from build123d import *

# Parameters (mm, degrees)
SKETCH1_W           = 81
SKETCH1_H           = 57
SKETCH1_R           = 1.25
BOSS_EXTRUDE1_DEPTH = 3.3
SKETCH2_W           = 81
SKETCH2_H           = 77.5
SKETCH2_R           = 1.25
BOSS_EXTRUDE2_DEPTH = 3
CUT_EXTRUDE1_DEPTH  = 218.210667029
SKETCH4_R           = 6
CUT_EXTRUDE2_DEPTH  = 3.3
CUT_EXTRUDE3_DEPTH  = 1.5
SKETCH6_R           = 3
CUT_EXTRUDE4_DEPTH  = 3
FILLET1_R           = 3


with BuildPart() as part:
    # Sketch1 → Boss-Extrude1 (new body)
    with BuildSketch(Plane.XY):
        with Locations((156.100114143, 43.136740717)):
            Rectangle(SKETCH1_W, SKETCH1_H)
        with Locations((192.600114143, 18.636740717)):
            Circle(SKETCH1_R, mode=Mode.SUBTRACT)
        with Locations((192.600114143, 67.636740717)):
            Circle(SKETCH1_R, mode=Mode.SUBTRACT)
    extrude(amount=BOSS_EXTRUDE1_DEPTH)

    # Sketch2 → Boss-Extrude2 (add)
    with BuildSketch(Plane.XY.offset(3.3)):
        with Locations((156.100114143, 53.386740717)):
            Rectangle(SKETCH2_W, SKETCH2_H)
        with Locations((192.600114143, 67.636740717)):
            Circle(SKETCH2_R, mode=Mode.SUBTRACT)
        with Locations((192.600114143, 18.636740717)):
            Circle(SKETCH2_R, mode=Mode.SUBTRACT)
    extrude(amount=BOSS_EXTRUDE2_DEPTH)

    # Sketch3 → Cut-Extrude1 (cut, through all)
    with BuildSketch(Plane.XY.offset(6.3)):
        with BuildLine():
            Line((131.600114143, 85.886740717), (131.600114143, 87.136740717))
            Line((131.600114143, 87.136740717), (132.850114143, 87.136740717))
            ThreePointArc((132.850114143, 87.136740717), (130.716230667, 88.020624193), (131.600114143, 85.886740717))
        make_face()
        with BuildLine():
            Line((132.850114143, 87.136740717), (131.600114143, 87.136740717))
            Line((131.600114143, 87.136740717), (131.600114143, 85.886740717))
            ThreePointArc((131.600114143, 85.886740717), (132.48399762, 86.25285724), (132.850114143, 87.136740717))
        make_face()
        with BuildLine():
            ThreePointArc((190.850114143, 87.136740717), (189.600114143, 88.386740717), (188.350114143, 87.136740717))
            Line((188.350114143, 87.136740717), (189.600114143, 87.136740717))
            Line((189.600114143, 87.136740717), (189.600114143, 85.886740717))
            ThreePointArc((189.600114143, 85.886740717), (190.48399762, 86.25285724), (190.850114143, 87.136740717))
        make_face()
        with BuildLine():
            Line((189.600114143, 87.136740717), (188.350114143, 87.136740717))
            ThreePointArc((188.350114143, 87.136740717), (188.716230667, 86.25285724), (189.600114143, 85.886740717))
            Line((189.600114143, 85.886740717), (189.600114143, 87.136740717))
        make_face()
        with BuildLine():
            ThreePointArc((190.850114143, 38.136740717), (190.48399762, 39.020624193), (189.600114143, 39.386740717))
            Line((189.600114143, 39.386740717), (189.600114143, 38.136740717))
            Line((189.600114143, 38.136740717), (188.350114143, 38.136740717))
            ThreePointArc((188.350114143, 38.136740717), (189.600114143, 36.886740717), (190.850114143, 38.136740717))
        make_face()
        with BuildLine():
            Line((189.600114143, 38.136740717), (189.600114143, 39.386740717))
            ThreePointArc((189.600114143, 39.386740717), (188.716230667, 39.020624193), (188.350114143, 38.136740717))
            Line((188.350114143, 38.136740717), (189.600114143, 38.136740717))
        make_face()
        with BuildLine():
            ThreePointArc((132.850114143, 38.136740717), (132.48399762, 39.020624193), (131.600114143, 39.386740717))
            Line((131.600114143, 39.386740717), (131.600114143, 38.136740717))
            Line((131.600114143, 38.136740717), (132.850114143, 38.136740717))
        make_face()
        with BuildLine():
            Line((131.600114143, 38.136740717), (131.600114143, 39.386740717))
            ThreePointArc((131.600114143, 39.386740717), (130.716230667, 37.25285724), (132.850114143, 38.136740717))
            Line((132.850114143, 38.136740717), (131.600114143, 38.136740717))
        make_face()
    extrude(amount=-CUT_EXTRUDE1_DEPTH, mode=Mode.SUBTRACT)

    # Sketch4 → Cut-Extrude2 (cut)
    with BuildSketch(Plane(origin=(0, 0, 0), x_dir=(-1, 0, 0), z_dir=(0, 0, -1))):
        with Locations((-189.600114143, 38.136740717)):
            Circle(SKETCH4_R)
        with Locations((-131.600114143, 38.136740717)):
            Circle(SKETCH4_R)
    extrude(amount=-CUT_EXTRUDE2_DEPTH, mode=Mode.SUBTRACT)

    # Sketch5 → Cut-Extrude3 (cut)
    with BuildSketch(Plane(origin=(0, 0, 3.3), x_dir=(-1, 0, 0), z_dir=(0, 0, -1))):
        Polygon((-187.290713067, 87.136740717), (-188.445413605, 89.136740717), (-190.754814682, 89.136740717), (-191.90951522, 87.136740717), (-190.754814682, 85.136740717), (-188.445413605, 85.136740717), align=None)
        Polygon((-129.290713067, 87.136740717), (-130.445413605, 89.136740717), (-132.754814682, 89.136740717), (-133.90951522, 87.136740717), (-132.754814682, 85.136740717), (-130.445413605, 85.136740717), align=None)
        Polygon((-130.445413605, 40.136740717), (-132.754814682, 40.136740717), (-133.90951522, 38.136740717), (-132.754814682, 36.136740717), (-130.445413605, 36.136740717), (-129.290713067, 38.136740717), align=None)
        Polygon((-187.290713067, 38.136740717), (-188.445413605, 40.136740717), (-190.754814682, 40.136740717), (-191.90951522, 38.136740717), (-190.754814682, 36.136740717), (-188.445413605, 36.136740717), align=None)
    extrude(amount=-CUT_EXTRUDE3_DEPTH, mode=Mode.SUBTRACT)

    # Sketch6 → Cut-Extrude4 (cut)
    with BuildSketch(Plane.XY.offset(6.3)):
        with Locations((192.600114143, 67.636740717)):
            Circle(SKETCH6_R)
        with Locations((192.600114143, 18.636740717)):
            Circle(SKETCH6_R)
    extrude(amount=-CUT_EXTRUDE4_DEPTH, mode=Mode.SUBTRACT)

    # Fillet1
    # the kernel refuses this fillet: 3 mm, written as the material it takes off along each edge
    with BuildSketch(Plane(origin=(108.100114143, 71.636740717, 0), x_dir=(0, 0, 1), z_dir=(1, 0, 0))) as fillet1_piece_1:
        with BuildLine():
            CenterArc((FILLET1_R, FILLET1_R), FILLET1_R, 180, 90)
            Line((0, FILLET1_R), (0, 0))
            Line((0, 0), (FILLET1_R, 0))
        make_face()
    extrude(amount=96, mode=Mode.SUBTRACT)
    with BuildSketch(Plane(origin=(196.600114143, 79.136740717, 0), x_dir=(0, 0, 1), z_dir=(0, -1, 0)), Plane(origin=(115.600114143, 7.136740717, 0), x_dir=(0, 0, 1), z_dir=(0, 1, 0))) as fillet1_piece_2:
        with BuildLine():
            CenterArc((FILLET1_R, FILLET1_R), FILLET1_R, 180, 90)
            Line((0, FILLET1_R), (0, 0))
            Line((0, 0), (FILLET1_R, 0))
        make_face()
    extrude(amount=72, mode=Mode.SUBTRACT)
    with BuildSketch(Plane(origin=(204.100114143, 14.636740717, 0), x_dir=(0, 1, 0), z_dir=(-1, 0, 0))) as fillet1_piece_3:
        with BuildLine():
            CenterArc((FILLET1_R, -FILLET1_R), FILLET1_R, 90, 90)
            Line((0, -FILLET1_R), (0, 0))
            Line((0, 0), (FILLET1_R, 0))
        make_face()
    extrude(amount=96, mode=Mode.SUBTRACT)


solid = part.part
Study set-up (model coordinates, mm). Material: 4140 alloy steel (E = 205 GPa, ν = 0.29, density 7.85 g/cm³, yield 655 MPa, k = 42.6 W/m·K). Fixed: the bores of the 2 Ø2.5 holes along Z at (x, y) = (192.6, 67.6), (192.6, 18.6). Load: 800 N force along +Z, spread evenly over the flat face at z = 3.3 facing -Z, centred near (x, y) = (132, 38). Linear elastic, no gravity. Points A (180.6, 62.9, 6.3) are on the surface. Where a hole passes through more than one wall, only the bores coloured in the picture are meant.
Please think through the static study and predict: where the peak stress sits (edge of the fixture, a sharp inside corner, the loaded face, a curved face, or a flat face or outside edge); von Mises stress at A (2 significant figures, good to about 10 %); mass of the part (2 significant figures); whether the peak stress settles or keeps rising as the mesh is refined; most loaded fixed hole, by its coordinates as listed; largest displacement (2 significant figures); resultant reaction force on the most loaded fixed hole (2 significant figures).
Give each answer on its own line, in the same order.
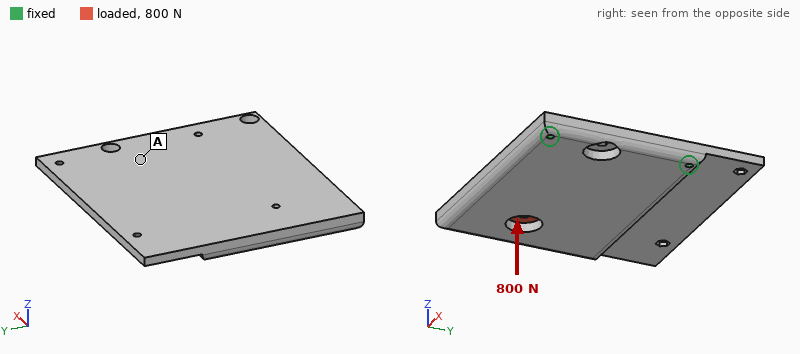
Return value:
edge of the fixture
98 MPa
260 g
keeps rising
(192.6, 18.6)
0.94 mm
530 N
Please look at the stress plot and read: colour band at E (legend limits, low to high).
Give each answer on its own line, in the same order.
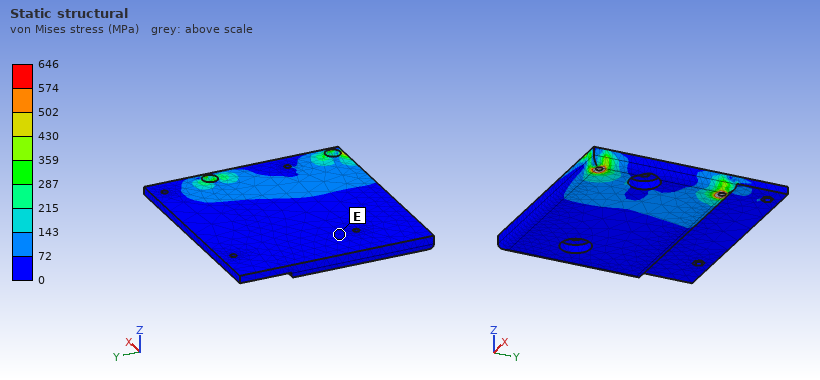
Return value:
0 to 72 MPa
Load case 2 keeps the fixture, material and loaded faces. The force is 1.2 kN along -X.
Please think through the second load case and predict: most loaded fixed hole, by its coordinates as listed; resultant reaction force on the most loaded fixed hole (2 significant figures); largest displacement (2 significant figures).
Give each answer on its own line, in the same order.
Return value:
(192.6, 18.6)
740 N
23 µm
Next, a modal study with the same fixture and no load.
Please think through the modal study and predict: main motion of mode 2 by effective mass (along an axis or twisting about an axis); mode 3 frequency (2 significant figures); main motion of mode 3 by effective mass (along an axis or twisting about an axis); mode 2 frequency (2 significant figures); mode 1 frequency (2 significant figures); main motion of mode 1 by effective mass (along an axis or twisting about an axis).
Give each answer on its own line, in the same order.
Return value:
twisting about X
3700 Hz
along Z
1800 Hz
480 Hz
along Z
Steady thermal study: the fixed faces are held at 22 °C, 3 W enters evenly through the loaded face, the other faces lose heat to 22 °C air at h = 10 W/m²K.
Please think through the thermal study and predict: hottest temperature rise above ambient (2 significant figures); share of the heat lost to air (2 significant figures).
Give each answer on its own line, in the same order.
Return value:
15 K
33 %
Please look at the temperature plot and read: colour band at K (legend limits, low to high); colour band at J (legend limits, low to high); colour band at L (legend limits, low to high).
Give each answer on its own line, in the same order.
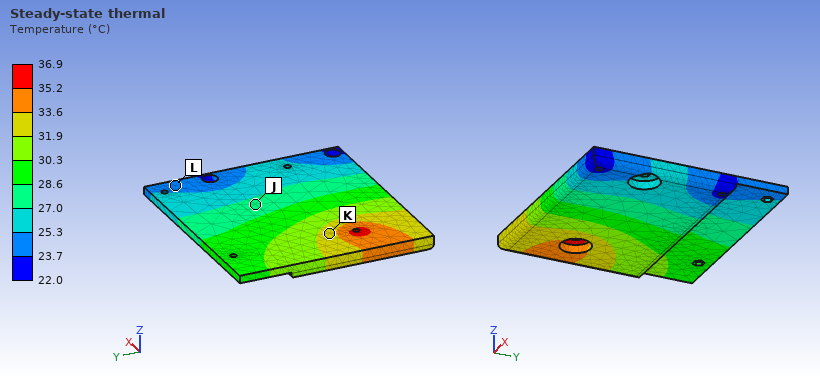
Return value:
31.9 to 33.6 °C
27.0 to 28.6 °C
23.7 to 25.3 °C
